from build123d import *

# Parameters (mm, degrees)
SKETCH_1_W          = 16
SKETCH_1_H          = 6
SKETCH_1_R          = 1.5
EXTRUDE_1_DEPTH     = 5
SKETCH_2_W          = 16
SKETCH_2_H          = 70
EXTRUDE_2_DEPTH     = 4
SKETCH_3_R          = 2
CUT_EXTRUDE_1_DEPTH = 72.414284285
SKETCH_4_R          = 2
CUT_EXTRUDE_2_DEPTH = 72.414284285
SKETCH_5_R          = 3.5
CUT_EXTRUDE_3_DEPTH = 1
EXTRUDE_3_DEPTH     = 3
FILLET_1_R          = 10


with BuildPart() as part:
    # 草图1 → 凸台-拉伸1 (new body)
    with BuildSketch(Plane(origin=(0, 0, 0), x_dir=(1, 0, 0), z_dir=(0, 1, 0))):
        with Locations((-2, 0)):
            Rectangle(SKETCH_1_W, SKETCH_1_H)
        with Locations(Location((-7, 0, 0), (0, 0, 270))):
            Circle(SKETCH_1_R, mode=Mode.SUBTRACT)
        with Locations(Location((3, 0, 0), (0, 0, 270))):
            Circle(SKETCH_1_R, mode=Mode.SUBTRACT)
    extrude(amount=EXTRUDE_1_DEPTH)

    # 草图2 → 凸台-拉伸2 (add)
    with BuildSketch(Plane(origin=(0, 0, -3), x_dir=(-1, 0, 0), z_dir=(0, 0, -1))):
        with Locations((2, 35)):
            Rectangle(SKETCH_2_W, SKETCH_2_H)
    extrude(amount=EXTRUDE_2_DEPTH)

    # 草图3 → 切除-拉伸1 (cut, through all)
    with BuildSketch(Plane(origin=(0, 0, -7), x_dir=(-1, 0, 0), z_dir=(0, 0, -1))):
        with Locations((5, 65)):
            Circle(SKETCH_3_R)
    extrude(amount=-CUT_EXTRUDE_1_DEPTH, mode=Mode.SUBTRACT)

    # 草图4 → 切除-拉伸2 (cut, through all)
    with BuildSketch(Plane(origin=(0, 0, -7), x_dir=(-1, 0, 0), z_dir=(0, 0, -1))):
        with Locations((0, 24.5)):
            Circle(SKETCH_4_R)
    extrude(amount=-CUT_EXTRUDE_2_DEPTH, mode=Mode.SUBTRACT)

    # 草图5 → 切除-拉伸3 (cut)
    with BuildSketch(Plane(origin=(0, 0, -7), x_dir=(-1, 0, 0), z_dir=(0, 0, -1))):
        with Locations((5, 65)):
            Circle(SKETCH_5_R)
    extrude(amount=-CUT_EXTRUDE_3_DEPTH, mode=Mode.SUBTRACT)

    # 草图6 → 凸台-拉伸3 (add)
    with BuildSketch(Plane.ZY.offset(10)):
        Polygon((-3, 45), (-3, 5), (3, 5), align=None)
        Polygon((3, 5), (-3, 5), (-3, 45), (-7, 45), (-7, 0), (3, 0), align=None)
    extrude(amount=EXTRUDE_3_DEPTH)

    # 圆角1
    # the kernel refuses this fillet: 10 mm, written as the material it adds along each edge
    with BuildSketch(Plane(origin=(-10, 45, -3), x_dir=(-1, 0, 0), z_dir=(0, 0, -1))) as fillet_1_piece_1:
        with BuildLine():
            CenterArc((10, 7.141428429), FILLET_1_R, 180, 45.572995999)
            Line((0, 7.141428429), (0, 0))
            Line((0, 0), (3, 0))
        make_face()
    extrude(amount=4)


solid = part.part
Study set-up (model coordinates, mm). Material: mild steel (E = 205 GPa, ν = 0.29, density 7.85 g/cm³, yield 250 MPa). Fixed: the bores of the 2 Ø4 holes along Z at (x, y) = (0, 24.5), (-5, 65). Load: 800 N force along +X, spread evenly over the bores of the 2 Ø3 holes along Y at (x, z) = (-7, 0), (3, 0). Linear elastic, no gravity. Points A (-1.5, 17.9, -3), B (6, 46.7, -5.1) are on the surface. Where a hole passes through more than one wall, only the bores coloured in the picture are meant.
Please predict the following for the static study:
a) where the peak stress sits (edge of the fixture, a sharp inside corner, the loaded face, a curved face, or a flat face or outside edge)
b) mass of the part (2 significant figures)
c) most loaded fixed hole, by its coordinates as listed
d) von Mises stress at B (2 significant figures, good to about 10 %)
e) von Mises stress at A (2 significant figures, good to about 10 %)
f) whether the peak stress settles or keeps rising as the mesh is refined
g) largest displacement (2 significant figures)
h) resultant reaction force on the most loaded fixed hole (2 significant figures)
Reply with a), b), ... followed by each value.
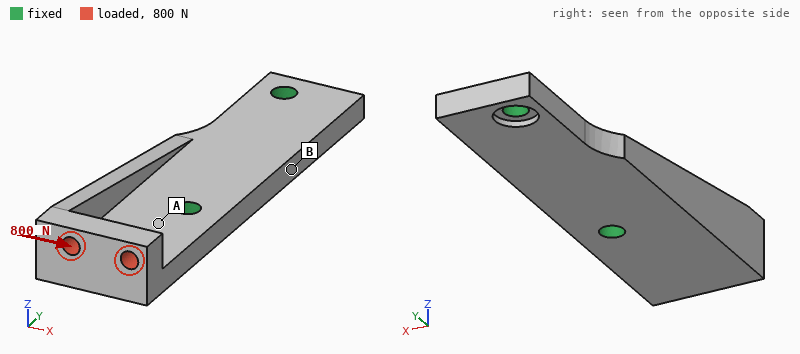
a) edge of the fixture
b) 45 g
c) (0, 24.5)
d) 17 MPa
e) 92 MPa
f) keeps rising
g) 49 µm
h) 1.1 kN
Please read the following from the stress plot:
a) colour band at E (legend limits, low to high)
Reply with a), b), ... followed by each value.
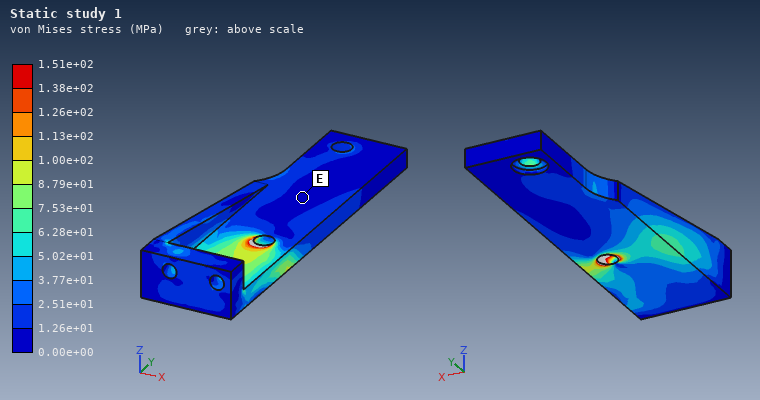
a) 0.00e+00 to 1.26e+01 MPa
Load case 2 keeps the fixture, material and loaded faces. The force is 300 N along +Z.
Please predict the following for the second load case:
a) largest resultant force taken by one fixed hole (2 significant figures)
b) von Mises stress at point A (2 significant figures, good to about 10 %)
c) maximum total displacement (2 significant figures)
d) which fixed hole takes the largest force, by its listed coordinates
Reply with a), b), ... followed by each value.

a) 350 N
b) 59 MPa
c) 46 µm
d) (0, 24.5)
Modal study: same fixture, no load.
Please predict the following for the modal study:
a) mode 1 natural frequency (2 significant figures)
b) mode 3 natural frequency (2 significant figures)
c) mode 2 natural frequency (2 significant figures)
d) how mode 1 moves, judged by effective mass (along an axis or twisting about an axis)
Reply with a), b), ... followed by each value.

a) 4400 Hz
b) 11 kHz
c) 8400 Hz
d) along Z
